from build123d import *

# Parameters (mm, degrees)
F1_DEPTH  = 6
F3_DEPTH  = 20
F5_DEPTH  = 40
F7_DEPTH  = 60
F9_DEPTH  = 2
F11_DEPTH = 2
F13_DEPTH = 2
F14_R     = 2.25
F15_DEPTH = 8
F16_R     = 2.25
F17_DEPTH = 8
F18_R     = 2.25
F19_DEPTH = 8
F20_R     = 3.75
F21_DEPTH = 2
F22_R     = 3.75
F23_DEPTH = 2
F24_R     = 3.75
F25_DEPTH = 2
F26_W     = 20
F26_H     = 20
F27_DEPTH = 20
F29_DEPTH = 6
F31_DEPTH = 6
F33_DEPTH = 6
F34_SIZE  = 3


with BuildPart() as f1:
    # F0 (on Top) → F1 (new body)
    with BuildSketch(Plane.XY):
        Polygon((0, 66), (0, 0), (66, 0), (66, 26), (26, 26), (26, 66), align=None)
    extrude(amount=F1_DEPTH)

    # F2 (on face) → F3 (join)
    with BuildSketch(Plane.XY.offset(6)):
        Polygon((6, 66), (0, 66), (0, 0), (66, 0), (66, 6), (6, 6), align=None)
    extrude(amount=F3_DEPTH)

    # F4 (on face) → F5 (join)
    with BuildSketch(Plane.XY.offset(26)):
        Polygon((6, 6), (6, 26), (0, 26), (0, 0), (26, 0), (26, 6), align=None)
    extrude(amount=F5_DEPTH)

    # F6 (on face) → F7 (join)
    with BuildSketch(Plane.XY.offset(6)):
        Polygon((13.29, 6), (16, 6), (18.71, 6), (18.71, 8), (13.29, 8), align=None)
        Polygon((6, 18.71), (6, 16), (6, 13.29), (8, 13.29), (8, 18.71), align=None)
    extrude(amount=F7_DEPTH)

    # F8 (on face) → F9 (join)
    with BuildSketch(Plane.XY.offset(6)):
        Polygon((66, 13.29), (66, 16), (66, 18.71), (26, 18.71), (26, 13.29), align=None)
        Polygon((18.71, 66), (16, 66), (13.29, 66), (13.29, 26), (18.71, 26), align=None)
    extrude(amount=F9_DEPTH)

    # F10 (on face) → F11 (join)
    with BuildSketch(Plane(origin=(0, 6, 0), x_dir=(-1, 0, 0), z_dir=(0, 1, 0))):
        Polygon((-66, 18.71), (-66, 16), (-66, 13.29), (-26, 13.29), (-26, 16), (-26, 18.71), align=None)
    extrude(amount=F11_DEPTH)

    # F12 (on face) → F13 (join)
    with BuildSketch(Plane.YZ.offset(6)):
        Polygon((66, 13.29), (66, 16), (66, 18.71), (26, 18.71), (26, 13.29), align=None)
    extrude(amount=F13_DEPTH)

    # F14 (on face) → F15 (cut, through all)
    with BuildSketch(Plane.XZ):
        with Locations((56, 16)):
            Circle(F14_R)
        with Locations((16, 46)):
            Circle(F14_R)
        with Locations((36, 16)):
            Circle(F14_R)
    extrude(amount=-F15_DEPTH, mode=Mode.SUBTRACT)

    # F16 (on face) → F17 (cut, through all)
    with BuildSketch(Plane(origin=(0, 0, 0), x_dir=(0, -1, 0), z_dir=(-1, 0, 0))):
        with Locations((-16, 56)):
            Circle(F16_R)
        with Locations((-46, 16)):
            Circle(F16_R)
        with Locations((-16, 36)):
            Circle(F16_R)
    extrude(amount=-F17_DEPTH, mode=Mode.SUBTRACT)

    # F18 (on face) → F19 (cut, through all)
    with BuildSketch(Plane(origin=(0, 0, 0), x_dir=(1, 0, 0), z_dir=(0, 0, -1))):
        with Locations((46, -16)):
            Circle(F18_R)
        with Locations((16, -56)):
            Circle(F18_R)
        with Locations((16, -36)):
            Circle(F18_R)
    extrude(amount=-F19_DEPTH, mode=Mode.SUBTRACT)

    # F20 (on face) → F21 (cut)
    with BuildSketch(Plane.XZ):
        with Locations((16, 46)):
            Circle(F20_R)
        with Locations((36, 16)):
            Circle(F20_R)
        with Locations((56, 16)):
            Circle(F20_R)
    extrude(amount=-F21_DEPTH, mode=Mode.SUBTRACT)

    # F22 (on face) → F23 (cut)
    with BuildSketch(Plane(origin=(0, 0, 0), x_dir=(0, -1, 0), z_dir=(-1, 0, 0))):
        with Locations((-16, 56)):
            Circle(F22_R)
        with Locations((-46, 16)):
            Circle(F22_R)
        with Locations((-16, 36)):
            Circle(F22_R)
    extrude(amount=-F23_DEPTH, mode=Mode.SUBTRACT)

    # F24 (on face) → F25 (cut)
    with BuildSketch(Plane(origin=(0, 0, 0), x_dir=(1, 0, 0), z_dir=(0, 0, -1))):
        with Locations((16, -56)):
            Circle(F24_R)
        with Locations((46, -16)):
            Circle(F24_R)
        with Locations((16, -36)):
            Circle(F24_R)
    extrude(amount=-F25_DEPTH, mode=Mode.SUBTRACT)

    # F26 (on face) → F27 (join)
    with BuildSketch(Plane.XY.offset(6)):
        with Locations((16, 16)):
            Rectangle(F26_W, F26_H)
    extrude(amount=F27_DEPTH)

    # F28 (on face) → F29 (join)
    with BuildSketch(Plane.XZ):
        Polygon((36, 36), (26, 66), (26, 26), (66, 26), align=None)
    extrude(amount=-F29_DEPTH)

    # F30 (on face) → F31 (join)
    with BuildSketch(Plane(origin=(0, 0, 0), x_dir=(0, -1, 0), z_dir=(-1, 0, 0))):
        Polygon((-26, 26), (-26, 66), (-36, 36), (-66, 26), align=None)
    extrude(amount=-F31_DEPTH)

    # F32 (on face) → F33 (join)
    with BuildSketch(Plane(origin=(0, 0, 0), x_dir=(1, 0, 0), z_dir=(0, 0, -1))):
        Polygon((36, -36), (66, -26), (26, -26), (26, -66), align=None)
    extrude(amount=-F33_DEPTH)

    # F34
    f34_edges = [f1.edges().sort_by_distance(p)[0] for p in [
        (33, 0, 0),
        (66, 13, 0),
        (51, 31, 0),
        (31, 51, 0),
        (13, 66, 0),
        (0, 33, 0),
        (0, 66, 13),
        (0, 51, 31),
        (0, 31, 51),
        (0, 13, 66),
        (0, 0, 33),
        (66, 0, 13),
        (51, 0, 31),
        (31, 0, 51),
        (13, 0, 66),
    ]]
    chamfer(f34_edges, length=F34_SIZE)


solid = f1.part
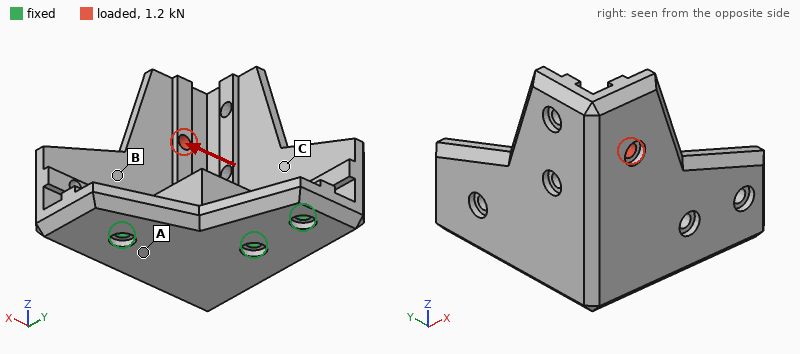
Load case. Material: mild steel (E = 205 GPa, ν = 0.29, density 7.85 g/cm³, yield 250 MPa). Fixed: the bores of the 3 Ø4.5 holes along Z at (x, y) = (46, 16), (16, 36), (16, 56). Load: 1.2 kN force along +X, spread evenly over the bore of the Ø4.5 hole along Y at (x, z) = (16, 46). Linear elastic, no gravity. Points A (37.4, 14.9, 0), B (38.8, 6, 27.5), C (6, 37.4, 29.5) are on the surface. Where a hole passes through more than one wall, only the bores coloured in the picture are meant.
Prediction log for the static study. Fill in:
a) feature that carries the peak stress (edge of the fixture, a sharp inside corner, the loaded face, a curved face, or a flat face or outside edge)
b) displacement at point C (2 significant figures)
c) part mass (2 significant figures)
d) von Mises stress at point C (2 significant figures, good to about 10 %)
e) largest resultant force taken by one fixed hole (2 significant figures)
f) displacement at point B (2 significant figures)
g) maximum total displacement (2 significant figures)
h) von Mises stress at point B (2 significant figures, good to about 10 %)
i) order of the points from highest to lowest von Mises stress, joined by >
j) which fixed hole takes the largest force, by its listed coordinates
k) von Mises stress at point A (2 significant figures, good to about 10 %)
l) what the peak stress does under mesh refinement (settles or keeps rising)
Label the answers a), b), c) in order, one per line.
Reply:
a) edge of the fixture
b) 24 µm
c) 440 g
d) 9.0 MPa
e) 1.9 kN
f) 22 µm
g) 71 µm
h) 17 MPa
i) A > B > C
j) (16, 36)
k) 29 MPa
l) keeps rising
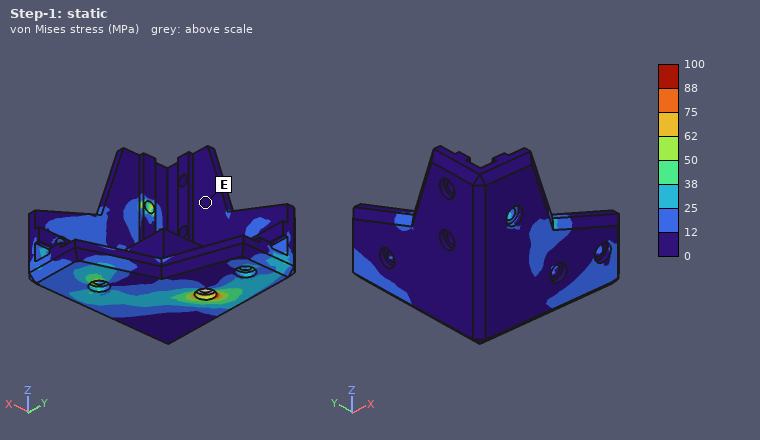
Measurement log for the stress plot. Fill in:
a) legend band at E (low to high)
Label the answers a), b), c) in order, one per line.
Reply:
a) 0 to 12 MPa
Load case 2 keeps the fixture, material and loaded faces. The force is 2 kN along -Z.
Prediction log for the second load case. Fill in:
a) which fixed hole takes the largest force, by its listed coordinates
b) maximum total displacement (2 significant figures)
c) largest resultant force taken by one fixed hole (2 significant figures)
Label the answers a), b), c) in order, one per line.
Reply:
a) (16, 36)
b) 86 µm
c) 2.8 kN
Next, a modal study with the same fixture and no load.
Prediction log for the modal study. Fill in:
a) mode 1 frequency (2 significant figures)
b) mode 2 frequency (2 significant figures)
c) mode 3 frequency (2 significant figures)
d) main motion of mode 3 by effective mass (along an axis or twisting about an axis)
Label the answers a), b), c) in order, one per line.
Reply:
a) 1600 Hz
b) 3600 Hz
c) 6500 Hz
d) along Z
